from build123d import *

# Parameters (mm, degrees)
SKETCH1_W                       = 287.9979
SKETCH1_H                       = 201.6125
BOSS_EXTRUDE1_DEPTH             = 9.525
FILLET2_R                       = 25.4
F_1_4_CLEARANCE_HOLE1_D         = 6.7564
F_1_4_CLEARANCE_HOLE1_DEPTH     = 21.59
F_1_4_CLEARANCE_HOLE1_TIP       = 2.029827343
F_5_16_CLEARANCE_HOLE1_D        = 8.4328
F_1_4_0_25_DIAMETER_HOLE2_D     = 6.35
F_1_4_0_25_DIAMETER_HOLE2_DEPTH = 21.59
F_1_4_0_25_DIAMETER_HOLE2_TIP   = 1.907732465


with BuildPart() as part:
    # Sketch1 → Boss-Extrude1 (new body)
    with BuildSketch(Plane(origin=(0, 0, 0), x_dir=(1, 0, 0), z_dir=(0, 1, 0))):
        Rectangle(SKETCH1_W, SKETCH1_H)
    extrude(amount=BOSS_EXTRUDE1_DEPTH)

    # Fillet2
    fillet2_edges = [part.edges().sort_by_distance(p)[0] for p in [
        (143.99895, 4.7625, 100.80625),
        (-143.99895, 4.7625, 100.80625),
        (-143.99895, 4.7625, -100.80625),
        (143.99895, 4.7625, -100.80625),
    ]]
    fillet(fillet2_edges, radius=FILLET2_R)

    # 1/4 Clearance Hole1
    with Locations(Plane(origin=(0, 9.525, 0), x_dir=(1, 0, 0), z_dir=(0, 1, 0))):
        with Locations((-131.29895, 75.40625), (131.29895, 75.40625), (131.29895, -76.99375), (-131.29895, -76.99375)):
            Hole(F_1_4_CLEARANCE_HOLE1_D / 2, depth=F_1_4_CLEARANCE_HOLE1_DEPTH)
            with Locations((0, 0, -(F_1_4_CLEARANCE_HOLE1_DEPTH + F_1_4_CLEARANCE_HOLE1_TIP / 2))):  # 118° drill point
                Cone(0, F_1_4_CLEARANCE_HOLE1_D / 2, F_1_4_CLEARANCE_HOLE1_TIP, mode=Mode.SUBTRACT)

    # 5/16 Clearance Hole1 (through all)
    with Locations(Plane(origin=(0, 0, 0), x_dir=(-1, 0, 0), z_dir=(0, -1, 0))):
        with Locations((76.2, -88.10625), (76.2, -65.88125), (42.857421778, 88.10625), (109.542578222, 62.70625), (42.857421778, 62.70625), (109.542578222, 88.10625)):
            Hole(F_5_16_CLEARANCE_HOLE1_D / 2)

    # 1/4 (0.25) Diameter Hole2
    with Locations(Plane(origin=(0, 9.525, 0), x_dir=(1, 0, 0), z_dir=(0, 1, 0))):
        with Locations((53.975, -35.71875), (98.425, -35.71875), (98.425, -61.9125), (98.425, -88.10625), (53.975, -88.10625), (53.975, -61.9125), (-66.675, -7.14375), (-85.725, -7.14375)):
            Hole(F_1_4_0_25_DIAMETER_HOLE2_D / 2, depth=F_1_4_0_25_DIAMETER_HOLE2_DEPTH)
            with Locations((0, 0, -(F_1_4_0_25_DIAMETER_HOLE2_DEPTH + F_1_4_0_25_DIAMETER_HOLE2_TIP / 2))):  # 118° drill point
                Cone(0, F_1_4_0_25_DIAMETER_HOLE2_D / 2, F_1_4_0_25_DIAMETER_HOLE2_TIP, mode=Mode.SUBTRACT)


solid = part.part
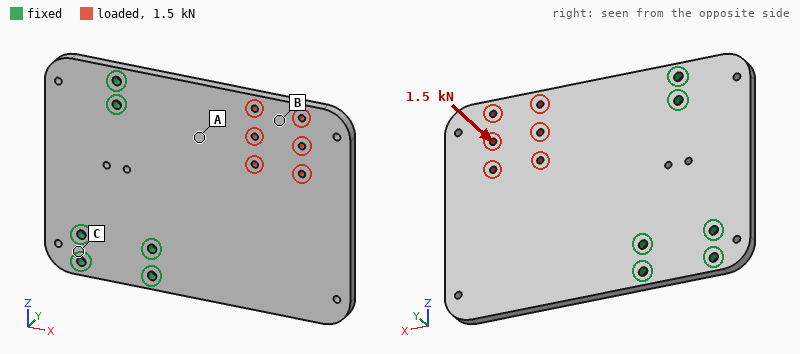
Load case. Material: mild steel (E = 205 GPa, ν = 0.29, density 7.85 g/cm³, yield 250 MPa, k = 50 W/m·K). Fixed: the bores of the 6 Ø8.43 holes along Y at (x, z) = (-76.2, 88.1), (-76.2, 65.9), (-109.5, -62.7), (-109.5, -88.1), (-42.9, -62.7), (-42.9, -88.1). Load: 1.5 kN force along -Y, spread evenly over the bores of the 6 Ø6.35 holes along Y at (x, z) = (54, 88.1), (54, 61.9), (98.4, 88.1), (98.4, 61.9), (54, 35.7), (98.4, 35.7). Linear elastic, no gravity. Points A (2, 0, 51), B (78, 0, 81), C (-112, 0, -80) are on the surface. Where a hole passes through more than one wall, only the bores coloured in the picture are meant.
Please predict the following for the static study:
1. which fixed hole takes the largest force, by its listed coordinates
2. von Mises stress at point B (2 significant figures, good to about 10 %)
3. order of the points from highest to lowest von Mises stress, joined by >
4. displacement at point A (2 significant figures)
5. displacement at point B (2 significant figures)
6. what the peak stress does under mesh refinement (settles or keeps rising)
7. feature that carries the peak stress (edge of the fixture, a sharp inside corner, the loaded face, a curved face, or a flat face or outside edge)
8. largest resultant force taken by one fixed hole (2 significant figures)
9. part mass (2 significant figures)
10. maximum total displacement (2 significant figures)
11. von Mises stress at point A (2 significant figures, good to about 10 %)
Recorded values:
(-42.9, -62.7)
18 MPa
A > B > C
0.20 mm
0.65 mm
keeps rising
edge of the fixture
2.3 kN
4.2 kg
1.0 mm
41 MPa
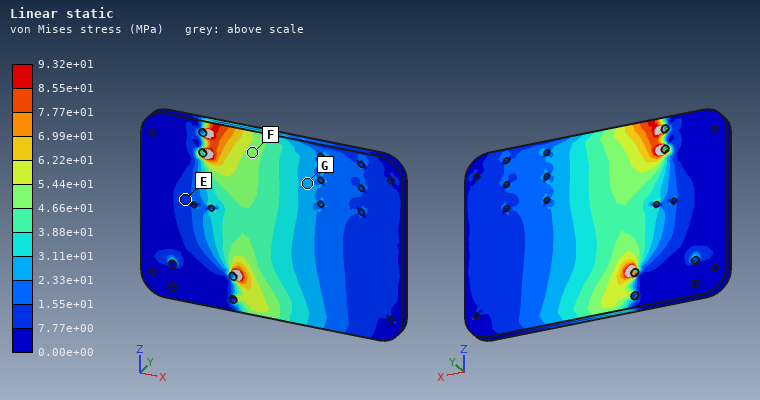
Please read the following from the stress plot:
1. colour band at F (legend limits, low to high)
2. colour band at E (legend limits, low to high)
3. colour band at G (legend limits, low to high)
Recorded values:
4.66e+01 to 5.44e+01 MPa
7.77e+00 to 1.55e+01 MPa
2.33e+01 to 3.11e+01 MPa
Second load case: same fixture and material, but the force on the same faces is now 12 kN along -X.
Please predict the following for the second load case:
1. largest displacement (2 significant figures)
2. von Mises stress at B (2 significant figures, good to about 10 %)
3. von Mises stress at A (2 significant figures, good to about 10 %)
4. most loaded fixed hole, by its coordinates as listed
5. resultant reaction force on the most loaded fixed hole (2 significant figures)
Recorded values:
18 µm
7.9 MPa
12 MPa
(-76.2, 65.9)
5.6 kN
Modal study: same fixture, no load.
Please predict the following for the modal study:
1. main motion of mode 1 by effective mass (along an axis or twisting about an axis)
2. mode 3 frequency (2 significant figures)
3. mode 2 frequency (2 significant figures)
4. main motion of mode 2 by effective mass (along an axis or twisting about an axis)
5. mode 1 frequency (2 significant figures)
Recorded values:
along Y
1100 Hz
500 Hz
twisting about X
190 Hz
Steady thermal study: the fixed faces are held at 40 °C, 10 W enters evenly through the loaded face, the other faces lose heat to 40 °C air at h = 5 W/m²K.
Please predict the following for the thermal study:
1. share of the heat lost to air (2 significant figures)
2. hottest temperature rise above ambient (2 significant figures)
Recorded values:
34 %
16 K
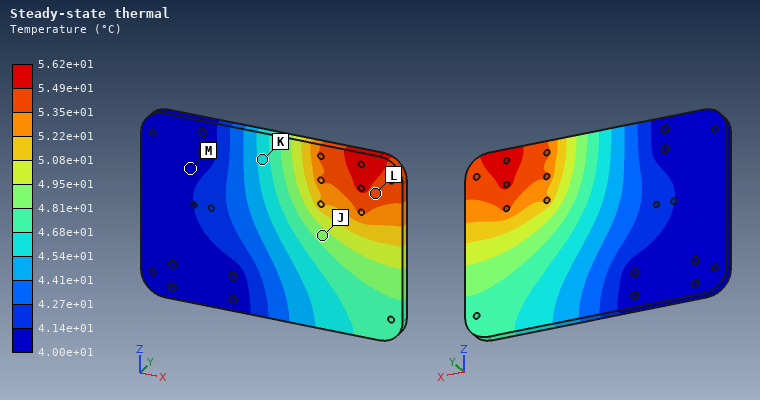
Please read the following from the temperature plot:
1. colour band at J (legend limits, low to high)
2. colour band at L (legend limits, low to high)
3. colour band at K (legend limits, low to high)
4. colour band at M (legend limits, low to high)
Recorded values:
4.81e+01 to 4.95e+01 °C
5.35e+01 to 5.49e+01 °C
4.54e+01 to 4.68e+01 °C
4.00e+01 to 4.14e+01 °C
